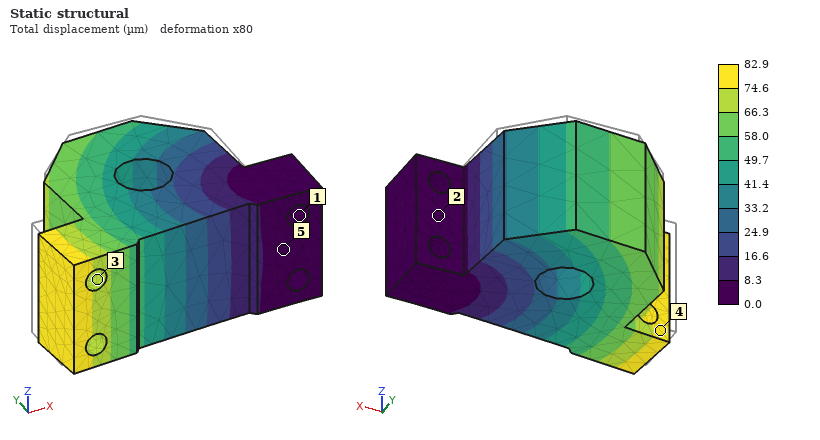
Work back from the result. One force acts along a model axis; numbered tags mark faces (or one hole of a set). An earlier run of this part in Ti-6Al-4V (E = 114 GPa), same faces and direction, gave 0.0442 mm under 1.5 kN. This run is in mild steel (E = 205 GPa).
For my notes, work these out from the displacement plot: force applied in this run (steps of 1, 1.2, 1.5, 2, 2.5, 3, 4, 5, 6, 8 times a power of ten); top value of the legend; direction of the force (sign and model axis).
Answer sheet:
5 kN
82.9 µm
-Y
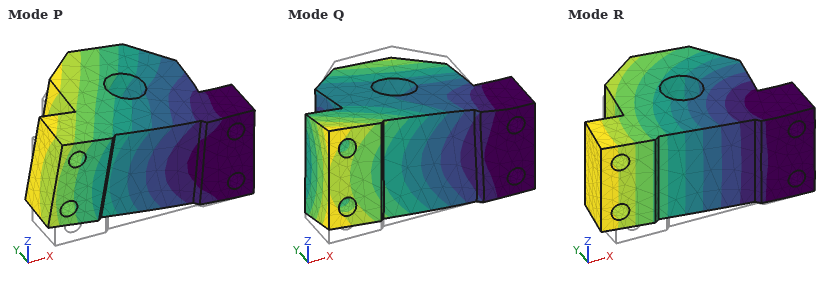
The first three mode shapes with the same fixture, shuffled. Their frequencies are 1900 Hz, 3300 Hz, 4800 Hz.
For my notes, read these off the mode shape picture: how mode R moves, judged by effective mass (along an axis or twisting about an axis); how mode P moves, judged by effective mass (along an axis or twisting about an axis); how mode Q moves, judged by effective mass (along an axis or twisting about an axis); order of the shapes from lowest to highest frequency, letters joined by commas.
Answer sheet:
along Y
along Z
twisting about X
R, P, Q
